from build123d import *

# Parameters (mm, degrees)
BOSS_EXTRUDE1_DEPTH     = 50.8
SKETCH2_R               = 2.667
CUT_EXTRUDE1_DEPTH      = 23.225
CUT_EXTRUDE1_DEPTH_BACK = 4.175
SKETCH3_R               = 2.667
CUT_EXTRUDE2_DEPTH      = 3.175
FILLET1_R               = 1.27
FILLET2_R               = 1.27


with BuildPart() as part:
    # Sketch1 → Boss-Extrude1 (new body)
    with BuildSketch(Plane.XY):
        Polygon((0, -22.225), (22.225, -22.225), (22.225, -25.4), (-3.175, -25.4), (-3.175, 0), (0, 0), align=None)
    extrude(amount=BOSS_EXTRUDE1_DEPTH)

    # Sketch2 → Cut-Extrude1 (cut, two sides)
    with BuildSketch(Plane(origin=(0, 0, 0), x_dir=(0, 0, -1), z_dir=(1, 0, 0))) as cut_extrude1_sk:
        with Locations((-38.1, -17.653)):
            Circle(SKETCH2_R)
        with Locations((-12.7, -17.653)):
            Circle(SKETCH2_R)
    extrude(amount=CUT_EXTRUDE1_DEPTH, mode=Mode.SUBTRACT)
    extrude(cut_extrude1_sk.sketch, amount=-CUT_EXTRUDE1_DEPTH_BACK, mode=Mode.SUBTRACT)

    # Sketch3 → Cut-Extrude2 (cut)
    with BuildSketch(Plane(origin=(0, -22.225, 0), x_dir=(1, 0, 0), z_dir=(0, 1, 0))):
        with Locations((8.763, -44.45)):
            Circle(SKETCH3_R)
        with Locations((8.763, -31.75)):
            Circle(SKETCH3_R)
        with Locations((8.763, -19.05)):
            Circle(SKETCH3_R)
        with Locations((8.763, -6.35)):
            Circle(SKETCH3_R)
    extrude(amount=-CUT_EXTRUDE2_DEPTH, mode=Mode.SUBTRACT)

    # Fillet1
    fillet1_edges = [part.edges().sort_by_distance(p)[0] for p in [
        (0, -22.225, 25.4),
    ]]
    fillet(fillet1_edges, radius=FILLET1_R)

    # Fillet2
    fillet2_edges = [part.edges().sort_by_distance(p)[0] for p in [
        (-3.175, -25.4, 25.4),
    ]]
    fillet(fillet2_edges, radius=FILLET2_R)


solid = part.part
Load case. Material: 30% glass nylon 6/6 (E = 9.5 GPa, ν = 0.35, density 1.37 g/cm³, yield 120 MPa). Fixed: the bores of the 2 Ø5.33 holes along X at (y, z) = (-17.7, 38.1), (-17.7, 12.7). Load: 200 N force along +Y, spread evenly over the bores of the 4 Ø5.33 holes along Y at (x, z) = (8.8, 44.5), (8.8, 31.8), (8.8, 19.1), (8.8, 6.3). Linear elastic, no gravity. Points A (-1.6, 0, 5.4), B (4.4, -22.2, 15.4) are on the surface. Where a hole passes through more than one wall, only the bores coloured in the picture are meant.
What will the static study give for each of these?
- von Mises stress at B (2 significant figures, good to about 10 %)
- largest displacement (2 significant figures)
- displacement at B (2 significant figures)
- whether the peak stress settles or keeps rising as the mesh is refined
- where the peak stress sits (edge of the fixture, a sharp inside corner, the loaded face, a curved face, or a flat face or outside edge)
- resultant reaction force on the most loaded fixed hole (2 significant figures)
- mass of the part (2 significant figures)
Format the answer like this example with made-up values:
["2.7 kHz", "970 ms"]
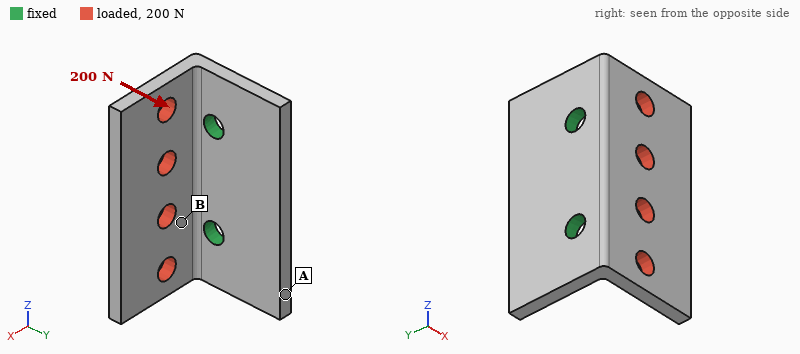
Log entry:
["9.7 MPa", "0.30 mm", "0.056 mm", "keeps rising", "edge of the fixture", "100 N", "9.9 g"]
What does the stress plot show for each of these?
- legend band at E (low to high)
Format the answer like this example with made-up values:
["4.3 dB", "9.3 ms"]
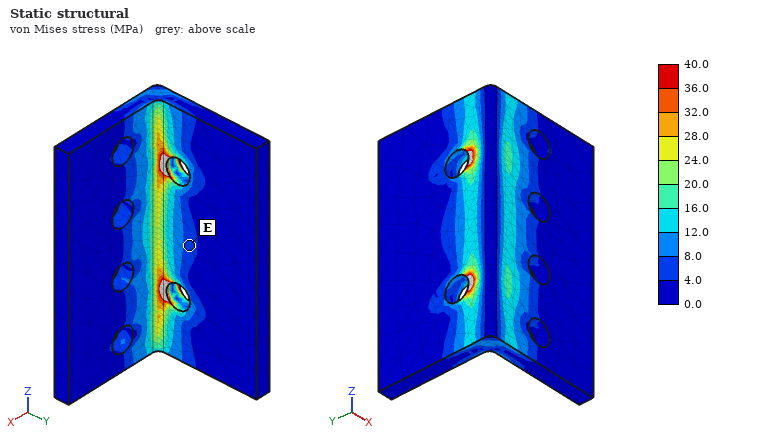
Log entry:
["4.0 to 8.0 MPa"]
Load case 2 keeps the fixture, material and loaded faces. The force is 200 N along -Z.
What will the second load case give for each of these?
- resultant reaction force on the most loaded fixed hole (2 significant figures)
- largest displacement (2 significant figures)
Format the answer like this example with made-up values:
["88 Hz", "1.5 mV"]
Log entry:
["130 N", "37 µm"]
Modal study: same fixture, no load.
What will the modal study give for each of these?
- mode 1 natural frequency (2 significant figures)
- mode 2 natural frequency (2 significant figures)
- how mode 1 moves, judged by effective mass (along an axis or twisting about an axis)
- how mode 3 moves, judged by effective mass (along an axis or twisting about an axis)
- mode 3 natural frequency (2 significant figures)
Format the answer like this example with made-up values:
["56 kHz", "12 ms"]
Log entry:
["1900 Hz", "2900 Hz", "along Y", "along X", "4600 Hz"]
